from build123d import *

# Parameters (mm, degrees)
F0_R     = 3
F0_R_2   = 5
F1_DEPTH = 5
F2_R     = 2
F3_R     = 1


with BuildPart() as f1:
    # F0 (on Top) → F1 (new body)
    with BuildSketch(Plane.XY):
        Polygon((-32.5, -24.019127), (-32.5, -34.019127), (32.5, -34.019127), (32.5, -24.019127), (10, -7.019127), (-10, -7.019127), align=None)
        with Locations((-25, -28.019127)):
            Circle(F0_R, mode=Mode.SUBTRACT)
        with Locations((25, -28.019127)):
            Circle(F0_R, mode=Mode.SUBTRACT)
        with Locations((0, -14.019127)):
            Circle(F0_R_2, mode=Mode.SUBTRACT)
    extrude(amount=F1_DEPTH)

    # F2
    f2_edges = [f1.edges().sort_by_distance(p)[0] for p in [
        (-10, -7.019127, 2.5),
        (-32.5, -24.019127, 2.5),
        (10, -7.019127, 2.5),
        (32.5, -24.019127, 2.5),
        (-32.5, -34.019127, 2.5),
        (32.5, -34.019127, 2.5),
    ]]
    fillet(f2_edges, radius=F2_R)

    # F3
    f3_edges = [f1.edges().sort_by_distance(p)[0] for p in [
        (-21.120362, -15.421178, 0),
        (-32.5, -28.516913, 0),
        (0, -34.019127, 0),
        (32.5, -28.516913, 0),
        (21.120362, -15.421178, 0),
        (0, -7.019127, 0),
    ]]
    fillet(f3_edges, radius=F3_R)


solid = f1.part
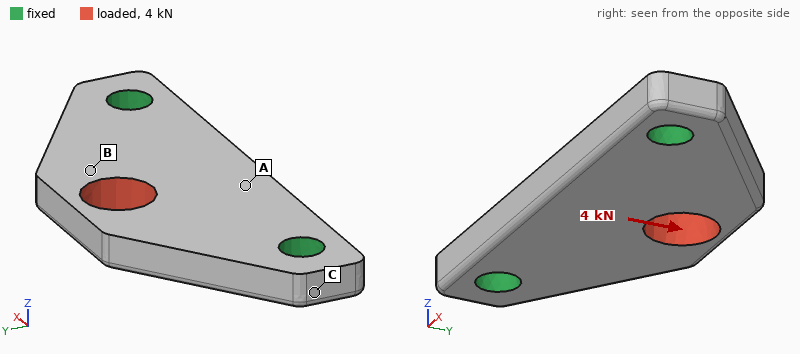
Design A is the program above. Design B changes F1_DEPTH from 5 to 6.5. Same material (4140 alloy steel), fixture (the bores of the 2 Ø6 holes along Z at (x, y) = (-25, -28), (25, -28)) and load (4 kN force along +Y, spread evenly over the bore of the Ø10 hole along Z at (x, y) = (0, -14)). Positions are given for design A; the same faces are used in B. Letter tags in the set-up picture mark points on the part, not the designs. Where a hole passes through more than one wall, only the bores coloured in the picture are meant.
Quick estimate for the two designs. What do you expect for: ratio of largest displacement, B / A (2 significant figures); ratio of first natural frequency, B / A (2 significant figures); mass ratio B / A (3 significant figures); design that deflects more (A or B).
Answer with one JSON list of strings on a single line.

["0.77", "1.2", "1.30", "A"]
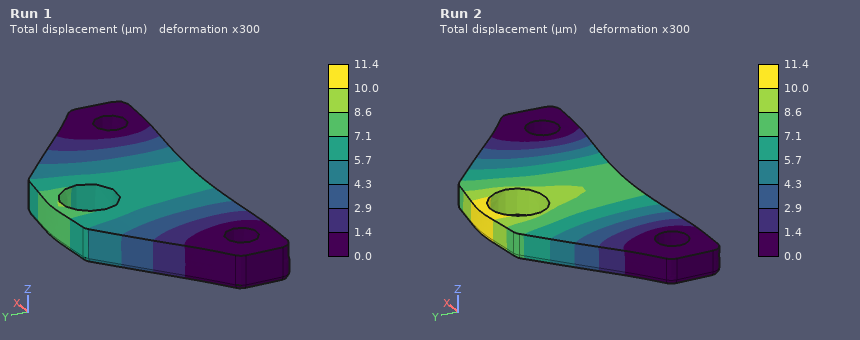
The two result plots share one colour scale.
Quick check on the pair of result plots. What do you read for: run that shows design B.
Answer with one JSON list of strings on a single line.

["Run 1"]
